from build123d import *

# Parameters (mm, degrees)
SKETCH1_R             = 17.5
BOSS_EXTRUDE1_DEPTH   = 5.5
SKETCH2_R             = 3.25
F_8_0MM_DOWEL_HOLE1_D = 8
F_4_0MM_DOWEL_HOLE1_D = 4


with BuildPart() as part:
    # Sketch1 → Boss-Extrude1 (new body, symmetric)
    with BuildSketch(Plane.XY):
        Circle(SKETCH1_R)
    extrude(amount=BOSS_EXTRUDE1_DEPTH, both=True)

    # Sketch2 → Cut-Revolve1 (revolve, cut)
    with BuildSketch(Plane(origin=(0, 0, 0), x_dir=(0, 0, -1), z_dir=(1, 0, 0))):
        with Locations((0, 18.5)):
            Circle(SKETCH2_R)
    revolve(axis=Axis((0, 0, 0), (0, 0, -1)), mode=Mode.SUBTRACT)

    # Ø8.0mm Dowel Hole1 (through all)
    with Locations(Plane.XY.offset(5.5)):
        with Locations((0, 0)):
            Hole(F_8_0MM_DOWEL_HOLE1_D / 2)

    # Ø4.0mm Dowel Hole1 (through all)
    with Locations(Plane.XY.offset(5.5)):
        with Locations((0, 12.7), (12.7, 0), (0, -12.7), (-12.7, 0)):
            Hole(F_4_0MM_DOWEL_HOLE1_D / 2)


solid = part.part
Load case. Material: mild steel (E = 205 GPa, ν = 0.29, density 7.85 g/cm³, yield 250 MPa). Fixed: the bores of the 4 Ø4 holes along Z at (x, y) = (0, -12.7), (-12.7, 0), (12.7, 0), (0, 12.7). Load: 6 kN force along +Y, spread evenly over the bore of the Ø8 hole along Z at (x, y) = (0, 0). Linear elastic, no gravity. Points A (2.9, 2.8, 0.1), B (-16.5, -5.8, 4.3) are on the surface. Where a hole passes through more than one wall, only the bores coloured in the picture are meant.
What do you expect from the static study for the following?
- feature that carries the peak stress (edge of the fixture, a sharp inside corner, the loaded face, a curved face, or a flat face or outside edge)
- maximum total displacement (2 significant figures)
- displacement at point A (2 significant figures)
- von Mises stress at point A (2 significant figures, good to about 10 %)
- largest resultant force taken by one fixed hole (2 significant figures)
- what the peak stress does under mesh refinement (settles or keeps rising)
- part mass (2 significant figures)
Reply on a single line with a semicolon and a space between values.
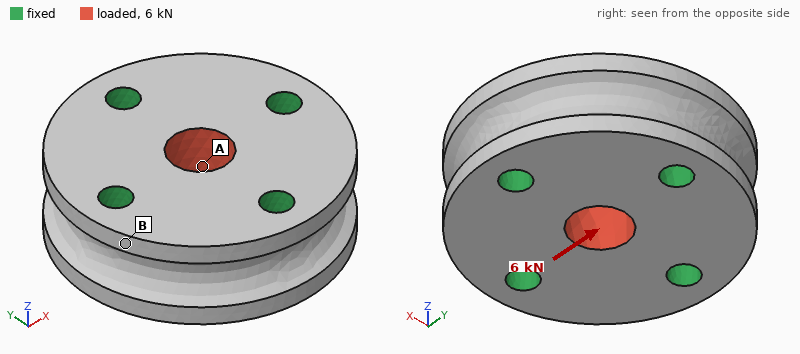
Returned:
edge of the fixture; 1.0 µm; 0.96 µm; 30 MPa; 2.0 kN; keeps rising; 66 g
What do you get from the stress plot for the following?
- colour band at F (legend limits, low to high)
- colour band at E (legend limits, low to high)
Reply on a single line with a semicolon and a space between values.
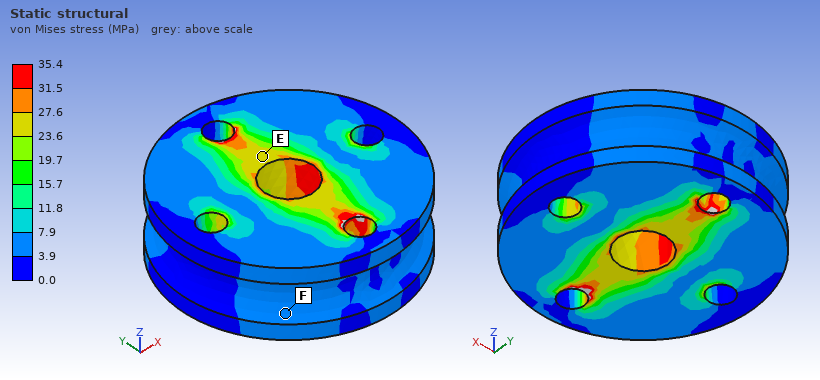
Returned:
3.9 to 7.9 MPa; 23.6 to 27.6 MPa
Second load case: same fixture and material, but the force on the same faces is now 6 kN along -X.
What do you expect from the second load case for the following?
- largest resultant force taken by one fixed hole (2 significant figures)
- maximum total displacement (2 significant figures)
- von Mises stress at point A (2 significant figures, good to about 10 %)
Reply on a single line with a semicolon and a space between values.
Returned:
2.0 kN; 1.0 µm; 29 MPa
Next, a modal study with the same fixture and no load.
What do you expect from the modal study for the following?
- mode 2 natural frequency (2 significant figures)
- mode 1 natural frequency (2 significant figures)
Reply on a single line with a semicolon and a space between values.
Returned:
66 kHz; 64 kHz
